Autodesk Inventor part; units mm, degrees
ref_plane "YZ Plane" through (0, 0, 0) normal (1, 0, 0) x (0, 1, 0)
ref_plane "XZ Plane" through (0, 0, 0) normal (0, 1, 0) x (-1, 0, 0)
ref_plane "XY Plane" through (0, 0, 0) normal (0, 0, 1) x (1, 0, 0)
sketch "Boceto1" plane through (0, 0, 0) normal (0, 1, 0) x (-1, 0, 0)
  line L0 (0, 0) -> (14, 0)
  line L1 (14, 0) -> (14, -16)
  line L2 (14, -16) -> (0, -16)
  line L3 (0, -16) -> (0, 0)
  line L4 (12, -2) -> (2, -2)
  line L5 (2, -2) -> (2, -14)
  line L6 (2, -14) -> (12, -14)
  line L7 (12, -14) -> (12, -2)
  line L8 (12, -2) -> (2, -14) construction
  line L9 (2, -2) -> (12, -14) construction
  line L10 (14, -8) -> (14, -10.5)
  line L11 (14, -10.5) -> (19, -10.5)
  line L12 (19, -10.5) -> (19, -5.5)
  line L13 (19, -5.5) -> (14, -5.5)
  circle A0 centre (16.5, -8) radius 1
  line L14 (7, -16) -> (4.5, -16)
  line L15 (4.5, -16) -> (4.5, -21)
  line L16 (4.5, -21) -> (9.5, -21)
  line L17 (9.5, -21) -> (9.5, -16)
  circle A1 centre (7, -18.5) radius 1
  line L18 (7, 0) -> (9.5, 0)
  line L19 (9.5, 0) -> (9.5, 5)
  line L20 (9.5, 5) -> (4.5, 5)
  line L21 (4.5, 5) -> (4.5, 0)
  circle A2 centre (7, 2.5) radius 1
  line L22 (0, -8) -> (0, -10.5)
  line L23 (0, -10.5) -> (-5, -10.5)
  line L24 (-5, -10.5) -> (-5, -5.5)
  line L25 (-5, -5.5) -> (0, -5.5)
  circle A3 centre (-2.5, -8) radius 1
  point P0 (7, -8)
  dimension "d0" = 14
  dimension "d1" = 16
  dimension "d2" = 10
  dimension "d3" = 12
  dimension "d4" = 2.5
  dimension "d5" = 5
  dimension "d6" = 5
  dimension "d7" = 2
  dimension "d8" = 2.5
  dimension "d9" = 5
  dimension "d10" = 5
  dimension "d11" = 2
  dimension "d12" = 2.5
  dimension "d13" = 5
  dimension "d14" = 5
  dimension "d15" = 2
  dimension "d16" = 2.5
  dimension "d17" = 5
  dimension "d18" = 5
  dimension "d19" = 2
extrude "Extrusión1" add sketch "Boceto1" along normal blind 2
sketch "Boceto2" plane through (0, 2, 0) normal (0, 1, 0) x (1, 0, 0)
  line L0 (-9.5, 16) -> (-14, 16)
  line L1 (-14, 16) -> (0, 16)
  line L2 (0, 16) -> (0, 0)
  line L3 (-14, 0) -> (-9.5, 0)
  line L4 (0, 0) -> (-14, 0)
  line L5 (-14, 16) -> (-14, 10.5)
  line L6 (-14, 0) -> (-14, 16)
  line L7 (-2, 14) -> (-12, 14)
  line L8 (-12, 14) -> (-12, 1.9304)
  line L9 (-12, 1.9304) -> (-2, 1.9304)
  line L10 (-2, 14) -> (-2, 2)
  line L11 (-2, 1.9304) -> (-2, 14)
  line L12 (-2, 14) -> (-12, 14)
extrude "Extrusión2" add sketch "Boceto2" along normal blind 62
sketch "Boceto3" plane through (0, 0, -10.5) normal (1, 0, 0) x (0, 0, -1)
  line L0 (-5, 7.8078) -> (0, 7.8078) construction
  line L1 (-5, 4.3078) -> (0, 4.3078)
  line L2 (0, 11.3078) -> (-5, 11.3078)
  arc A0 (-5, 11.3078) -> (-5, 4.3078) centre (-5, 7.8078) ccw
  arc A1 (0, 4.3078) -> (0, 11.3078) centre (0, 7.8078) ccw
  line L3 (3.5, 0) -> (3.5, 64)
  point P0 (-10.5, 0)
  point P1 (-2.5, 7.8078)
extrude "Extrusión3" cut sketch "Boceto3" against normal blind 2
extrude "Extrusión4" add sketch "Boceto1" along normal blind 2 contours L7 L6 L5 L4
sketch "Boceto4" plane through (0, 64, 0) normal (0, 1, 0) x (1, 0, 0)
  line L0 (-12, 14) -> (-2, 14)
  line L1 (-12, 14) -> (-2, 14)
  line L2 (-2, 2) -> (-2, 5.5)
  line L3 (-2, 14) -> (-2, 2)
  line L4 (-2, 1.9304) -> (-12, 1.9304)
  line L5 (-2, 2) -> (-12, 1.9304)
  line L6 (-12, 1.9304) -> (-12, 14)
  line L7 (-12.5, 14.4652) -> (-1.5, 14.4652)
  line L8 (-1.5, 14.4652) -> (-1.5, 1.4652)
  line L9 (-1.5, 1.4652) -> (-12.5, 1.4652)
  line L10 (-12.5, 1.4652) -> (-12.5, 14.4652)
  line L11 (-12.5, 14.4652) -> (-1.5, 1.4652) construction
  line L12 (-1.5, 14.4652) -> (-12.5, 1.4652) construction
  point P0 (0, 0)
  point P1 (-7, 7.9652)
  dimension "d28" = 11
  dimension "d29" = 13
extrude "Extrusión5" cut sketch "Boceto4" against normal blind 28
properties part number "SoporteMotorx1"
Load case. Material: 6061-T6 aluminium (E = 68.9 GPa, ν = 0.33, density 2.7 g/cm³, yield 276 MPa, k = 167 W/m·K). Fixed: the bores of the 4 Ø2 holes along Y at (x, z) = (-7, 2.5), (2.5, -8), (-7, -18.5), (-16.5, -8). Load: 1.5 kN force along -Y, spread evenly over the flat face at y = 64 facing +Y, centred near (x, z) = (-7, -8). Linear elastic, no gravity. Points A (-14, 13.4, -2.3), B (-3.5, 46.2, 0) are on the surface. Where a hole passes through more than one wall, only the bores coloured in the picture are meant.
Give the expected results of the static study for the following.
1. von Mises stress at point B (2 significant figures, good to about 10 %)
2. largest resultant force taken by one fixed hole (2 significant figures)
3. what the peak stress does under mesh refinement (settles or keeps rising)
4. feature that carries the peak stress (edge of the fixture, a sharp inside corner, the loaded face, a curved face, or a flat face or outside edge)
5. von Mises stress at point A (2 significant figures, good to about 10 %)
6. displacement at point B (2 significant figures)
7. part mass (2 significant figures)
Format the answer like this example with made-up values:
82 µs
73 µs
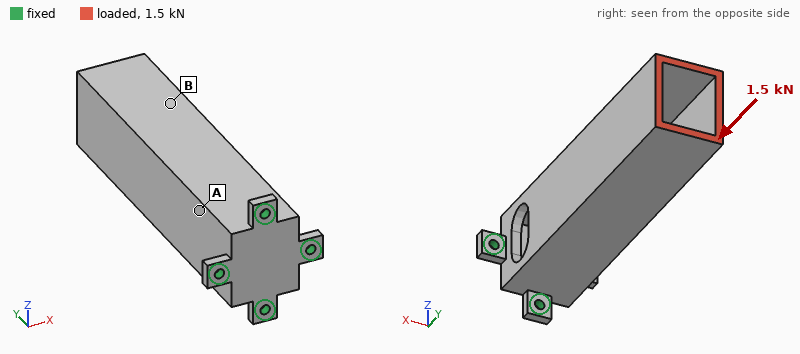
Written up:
19 MPa
470 N
keeps rising
edge of the fixture
11 MPa
39 µm
17 g
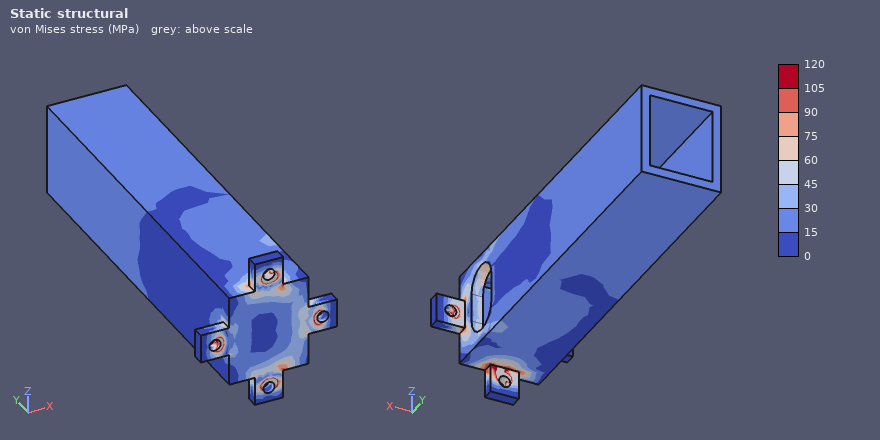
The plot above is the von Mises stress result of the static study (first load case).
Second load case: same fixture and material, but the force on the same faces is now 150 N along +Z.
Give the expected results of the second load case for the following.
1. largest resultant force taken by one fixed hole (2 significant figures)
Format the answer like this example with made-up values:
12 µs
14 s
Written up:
530 N
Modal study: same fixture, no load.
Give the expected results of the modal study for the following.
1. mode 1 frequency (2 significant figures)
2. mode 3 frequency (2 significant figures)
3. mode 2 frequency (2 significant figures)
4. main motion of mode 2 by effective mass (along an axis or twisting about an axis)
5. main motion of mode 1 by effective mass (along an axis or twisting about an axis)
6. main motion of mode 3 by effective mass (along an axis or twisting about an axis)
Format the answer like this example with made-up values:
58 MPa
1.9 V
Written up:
1800 Hz
8700 Hz
2300 Hz
along Z
along X
twisting about Y
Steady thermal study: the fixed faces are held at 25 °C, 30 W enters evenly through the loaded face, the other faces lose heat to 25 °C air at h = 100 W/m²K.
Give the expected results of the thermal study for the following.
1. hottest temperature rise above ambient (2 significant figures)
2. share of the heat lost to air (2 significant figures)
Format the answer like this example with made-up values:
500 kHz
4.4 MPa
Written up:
74 K
69 %
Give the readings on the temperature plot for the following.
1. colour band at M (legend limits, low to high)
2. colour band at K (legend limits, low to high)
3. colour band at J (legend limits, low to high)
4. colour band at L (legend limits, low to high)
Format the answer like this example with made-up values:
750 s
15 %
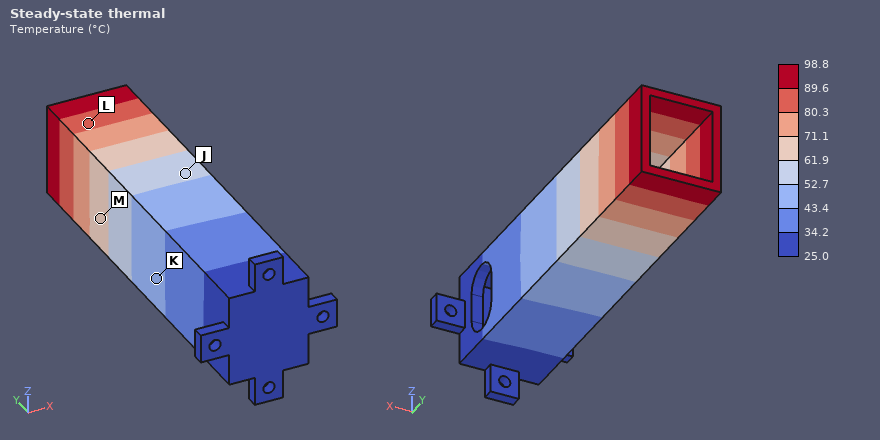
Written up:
61.9 to 71.1 °C
43.4 to 52.7 °C
52.7 to 61.9 °C
80.3 to 89.6 °C
